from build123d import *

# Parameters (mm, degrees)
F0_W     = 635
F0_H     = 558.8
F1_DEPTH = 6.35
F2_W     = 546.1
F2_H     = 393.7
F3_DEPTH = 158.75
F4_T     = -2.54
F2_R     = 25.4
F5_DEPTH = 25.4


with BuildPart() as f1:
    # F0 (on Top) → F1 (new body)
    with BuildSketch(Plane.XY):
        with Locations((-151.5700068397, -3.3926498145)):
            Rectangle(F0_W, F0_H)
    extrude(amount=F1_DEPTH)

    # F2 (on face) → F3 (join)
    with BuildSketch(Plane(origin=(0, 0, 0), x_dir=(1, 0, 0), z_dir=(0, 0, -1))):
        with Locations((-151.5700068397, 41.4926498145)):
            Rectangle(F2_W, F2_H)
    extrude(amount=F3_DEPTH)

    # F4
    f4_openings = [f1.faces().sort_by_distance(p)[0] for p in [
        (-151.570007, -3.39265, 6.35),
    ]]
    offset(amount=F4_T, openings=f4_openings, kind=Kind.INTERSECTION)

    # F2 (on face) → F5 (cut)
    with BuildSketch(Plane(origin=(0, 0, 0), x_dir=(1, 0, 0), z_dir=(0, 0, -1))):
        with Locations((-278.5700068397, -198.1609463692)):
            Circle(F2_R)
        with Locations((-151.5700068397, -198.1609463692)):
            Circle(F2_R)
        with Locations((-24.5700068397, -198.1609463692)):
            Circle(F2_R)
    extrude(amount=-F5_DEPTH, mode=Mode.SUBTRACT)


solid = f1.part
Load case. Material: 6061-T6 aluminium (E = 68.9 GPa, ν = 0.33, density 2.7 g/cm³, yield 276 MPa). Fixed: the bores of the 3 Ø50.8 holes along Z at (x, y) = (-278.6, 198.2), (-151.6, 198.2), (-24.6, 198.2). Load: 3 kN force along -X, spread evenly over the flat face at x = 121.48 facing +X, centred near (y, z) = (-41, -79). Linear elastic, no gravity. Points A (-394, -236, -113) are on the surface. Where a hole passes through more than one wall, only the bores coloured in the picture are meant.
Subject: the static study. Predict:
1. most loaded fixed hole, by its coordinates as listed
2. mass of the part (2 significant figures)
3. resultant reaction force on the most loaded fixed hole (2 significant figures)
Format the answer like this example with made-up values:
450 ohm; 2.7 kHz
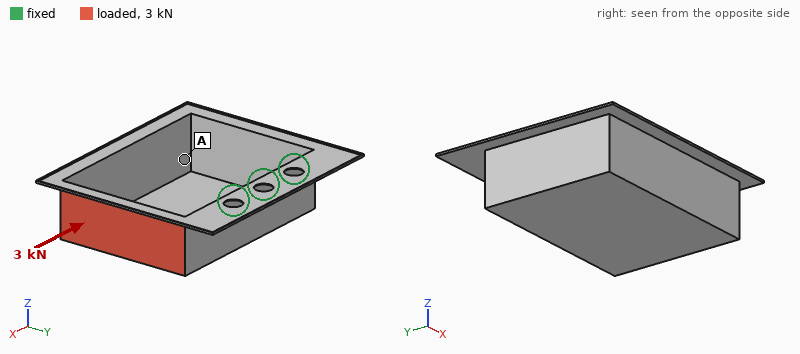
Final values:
(-24.6, 198.2); 4.5 kg; 2.5 kN
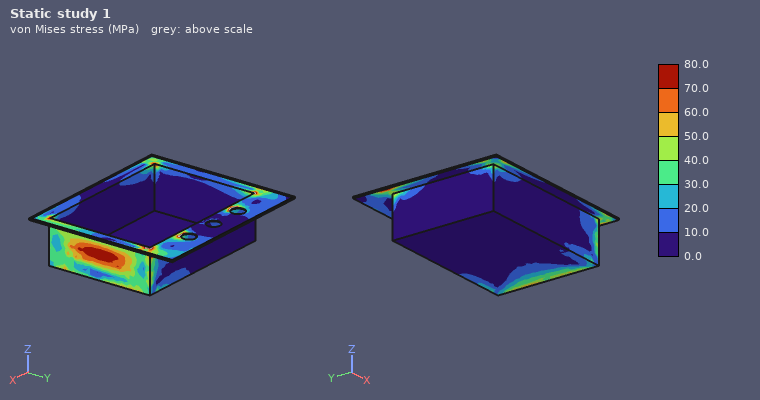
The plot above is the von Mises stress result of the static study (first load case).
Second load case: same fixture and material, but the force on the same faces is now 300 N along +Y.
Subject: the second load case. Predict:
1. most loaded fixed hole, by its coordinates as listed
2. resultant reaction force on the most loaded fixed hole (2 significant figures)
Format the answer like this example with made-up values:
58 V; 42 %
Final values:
(-24.6, 198.2); 410 N
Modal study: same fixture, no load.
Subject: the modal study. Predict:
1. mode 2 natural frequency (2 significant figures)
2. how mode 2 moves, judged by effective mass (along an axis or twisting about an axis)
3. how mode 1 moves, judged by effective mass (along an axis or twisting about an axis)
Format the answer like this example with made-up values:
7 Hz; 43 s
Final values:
79 Hz; along X; along Z
